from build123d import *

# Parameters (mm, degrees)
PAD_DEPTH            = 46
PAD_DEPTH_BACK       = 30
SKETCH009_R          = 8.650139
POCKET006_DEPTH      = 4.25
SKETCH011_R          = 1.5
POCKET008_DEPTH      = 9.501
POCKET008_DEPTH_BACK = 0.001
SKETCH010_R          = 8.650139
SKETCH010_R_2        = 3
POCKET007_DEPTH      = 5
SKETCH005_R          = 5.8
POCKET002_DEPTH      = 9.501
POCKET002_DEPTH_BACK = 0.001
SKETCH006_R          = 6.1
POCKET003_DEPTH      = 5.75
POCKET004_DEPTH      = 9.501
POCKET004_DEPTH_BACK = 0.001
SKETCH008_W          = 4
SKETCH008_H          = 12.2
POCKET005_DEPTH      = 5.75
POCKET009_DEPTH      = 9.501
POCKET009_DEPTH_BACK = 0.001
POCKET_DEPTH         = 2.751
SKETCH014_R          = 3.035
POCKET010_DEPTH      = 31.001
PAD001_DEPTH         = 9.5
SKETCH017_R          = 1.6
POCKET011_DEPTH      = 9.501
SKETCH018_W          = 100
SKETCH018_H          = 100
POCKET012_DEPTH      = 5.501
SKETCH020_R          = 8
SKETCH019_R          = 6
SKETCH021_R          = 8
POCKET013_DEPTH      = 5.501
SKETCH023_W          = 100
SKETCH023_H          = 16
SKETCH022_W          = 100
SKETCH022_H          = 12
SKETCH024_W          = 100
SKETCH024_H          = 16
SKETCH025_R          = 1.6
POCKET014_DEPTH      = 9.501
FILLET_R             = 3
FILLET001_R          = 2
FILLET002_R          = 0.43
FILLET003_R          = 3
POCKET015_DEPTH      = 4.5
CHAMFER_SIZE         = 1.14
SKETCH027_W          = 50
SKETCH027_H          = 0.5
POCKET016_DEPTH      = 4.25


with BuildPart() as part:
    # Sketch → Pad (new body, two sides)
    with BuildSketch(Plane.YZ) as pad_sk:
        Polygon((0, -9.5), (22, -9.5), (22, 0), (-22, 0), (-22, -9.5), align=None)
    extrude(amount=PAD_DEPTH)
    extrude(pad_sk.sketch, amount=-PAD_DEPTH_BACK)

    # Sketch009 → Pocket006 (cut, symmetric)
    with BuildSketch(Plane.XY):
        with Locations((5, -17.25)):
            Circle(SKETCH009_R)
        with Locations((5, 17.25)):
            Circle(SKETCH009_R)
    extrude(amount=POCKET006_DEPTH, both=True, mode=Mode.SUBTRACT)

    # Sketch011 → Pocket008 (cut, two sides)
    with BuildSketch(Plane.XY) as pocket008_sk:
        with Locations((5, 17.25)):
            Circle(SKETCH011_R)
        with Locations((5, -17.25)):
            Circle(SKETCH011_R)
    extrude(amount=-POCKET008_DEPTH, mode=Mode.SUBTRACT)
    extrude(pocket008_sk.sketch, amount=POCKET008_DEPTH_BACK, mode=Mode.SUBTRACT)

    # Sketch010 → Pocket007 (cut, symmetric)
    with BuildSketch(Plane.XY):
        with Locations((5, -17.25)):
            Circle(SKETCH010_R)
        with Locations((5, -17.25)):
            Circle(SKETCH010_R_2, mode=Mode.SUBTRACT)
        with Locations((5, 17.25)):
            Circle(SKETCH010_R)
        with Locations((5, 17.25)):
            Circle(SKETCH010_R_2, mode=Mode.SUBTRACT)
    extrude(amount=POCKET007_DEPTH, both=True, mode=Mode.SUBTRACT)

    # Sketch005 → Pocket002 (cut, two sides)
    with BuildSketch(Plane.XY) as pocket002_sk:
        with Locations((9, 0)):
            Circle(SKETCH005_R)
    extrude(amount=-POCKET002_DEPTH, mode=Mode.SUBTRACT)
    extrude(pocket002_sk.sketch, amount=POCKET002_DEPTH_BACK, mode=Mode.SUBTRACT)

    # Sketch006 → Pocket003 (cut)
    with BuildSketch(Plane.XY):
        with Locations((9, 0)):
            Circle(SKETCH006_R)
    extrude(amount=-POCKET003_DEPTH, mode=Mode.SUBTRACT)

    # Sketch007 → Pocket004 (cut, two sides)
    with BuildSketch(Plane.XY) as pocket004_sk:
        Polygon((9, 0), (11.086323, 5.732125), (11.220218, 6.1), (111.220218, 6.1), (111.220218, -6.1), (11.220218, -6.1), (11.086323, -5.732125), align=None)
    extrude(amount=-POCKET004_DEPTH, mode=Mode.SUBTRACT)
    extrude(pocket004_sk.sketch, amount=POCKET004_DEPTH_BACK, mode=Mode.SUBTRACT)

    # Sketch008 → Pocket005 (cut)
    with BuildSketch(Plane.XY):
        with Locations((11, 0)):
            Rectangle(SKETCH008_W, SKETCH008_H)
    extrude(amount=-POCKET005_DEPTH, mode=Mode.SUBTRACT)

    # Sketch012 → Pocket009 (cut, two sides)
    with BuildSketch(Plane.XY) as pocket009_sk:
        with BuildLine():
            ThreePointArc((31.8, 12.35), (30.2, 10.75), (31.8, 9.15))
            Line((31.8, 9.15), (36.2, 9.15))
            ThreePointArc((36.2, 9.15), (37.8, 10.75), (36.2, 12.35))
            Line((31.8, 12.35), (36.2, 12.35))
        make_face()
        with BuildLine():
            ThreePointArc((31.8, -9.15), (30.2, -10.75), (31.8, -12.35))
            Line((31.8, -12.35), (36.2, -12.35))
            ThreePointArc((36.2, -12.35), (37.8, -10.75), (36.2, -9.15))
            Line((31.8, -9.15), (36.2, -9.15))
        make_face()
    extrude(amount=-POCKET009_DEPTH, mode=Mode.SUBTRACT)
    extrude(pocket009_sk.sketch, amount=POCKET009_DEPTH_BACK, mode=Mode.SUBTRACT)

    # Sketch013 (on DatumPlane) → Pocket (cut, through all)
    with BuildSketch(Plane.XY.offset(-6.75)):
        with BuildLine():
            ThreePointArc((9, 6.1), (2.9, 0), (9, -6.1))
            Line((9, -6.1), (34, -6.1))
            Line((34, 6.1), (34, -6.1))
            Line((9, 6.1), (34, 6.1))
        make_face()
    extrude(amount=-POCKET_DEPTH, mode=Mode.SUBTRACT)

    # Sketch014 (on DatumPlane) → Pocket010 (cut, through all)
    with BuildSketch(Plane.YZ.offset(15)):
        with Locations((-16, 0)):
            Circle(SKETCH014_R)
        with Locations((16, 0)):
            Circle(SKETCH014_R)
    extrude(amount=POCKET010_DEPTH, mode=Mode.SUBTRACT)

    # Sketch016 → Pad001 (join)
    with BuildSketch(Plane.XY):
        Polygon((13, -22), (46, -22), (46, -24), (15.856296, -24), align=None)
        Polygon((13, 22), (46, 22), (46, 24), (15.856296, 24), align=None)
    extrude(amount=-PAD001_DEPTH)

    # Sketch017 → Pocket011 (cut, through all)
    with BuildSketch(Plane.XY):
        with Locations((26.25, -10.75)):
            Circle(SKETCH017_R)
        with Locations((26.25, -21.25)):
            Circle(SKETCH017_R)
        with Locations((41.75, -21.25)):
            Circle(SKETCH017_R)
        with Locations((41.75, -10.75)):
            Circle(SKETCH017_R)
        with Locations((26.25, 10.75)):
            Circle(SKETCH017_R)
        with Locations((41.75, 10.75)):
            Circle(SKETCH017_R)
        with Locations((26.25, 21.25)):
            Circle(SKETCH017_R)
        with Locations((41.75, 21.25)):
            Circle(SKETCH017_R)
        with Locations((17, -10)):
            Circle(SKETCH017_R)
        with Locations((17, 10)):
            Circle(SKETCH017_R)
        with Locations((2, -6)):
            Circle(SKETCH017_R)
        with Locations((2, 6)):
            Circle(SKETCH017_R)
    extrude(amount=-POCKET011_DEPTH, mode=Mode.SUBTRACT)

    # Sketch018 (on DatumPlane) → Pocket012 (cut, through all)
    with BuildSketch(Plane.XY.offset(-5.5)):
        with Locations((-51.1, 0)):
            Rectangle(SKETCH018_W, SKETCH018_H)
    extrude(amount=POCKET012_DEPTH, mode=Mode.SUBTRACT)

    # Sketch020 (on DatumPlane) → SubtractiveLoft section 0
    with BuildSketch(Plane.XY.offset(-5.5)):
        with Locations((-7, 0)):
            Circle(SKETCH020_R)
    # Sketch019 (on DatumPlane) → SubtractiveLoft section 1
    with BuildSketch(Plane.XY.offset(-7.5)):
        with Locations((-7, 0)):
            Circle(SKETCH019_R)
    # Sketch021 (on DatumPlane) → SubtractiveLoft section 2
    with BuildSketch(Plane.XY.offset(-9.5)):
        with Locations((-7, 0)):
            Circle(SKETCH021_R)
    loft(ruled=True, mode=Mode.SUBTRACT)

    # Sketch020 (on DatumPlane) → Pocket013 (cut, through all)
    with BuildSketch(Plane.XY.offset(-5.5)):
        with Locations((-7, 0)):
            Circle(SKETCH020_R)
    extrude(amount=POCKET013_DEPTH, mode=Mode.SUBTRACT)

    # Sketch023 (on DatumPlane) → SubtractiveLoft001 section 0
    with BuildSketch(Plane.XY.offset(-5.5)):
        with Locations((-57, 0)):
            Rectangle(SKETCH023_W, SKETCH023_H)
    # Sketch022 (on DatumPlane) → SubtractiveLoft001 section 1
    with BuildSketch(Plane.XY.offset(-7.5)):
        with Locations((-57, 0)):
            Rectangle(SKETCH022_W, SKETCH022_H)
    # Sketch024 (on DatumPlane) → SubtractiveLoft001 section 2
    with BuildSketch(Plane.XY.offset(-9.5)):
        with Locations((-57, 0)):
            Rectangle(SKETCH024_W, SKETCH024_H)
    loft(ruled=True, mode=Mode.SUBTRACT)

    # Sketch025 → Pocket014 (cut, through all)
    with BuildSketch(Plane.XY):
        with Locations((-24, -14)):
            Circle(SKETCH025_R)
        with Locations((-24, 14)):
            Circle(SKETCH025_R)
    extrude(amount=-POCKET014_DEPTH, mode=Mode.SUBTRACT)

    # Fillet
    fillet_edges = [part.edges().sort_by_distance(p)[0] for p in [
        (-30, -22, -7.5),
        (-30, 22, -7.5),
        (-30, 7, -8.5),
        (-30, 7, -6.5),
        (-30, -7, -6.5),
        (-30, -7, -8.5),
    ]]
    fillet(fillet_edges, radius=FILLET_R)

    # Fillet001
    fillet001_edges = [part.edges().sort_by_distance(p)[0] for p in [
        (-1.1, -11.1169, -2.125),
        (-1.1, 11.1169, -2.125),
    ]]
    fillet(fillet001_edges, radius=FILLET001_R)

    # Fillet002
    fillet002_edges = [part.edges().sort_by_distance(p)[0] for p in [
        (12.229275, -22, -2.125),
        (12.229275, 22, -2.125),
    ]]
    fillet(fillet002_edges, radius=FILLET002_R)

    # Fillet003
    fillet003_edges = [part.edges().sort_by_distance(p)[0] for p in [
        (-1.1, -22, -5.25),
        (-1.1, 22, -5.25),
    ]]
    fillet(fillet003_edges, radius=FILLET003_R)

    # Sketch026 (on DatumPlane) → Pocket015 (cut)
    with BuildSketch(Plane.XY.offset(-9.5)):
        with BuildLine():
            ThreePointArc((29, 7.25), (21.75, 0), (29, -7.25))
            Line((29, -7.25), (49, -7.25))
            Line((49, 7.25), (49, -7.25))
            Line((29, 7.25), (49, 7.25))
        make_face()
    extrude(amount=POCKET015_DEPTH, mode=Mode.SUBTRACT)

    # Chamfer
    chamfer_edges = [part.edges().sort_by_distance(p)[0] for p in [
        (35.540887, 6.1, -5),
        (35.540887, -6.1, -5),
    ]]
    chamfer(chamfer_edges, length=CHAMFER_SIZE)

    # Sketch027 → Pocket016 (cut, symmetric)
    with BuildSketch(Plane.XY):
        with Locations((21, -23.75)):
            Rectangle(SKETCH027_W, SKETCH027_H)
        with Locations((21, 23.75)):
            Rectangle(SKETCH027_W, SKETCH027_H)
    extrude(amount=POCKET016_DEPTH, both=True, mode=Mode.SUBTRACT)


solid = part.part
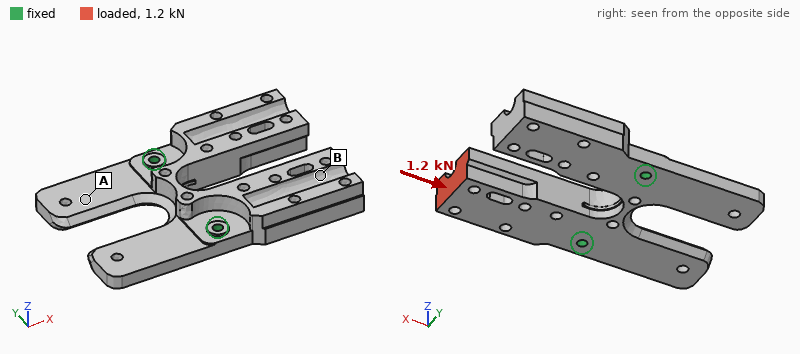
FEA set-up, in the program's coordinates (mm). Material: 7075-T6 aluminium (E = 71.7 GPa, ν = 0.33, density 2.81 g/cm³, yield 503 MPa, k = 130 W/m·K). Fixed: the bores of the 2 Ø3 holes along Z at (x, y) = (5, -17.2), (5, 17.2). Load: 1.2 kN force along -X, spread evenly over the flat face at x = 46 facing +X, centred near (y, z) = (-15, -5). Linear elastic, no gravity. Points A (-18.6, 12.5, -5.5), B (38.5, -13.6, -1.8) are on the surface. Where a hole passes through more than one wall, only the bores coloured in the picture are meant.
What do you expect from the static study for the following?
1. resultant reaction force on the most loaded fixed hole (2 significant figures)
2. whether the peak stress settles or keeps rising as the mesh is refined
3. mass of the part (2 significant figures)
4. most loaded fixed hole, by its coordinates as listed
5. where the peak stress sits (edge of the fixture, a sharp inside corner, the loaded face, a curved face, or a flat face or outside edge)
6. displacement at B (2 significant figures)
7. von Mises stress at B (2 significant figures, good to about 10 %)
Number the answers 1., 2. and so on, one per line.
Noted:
1. 1.1 kN
2. keeps rising
3. 42 g
4. (5, -17.2)
5. edge of the fixture
6. 56 µm
7. 15 MPa
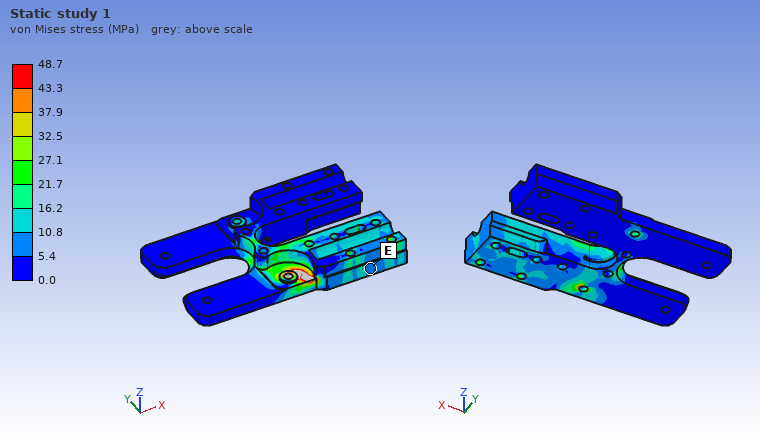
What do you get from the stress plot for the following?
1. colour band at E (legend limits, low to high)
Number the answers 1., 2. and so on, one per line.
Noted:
1. 5.4 to 10.8 MPa
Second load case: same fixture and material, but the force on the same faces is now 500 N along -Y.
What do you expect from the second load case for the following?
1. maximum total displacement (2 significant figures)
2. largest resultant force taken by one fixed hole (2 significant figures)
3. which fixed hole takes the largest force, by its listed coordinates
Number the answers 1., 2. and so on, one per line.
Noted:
1. 0.21 mm
2. 1.2 kN
3. (5, -17.2)
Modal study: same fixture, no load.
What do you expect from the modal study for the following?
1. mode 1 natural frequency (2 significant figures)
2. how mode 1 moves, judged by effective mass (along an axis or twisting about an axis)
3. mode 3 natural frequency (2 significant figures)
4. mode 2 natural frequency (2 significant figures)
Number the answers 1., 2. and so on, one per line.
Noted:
1. 2100 Hz
2. along Z
3. 3000 Hz
4. 2200 Hz
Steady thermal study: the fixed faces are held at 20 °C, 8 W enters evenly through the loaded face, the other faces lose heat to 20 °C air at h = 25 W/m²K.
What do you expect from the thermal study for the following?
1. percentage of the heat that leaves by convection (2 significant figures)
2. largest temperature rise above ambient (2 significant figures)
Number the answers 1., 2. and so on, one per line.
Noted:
1. 13 %
2. 23 K
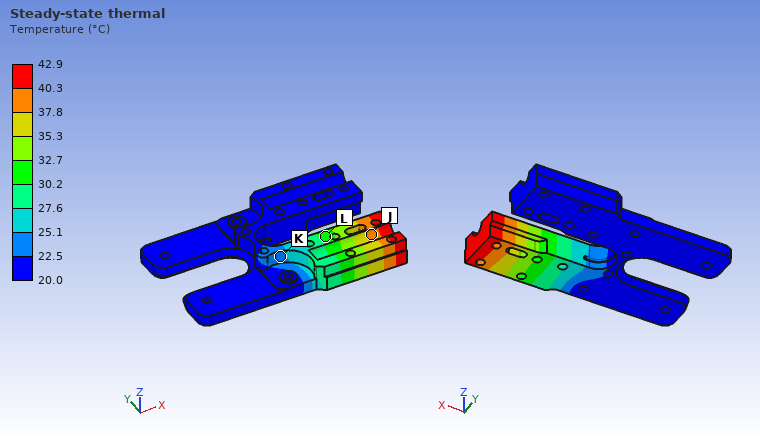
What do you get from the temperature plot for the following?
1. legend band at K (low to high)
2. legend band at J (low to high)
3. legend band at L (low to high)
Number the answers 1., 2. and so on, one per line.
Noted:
1. 22.5 to 25.1 °C
2. 37.8 to 40.3 °C
3. 30.2 to 32.7 °C
